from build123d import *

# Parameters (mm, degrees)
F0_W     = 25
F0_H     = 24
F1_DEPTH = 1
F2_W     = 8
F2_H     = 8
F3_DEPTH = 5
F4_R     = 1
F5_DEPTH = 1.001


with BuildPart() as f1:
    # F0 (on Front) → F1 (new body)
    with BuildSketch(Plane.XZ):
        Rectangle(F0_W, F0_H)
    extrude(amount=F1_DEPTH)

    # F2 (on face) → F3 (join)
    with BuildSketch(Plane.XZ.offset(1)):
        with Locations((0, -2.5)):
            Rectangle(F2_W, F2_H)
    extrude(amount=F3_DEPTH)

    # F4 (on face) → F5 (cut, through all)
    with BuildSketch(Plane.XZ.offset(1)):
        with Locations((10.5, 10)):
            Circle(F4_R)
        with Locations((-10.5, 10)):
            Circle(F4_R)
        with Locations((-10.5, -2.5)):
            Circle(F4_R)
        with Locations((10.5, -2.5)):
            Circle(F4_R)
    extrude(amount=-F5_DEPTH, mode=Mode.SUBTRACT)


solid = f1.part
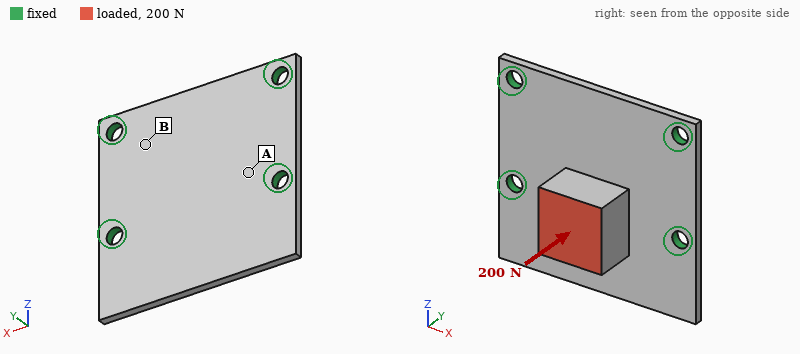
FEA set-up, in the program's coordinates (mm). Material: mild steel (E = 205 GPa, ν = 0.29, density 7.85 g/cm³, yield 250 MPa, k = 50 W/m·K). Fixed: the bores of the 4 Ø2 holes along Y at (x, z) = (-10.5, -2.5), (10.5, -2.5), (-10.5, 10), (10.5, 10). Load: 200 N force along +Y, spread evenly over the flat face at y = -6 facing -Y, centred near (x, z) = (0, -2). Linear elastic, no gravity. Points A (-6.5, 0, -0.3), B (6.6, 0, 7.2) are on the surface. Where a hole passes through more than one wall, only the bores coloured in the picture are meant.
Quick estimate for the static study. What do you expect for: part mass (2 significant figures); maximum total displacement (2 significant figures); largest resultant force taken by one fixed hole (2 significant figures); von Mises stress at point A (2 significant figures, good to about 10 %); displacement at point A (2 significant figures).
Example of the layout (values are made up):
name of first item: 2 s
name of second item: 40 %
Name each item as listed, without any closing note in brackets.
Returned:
part mass: 7.1 g
maximum total displacement: 25 µm
largest resultant force taken by one fixed hole: 100 N
von Mises stress at point A: 45 MPa
displacement at point A: 7.5 µm
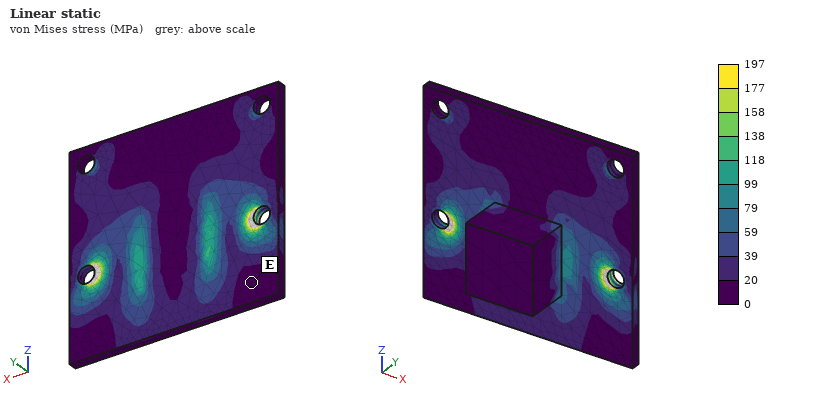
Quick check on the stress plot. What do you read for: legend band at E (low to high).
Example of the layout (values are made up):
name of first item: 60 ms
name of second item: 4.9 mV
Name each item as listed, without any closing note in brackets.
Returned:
legend band at E: 0 to 20 MPa
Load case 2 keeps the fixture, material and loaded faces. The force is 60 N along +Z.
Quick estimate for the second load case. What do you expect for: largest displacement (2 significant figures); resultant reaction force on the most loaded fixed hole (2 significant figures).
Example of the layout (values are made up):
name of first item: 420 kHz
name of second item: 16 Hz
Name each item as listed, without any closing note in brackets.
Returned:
largest displacement: 13 µm
resultant reaction force on the most loaded fixed hole: 21 N
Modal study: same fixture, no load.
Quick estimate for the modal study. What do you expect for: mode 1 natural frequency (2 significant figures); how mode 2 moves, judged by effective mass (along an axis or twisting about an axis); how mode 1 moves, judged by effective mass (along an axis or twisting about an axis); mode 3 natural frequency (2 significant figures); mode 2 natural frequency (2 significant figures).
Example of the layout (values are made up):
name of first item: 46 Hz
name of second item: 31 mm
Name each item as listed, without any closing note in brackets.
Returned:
mode 1 natural frequency: 7200 Hz
how mode 2 moves, judged by effective mass: along Y
how mode 1 moves, judged by effective mass: along Y
mode 3 natural frequency: 14 kHz
mode 2 natural frequency: 10 kHz
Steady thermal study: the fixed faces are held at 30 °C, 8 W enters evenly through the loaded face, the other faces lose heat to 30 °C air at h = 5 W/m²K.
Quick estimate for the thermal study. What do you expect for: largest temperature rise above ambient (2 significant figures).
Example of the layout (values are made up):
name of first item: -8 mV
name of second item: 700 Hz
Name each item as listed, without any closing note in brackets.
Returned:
largest temperature rise above ambient: 55 K
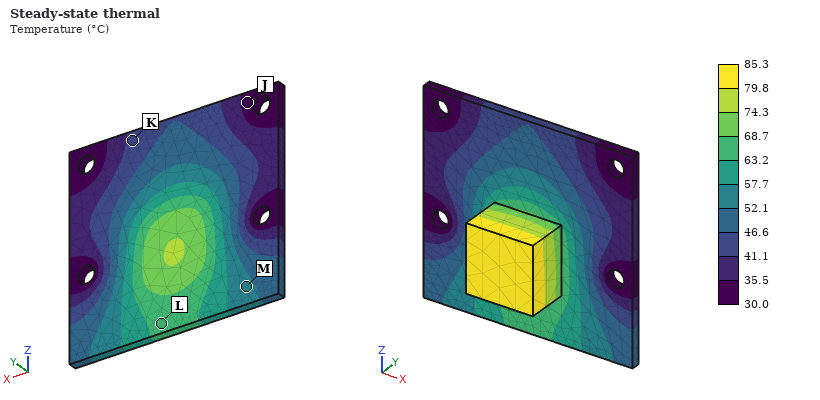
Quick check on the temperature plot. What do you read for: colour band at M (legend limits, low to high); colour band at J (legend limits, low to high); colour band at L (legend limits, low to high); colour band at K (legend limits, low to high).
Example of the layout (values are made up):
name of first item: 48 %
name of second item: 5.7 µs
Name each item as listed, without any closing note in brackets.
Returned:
colour band at M: 52.1 to 57.7 °C
colour band at J: 30.0 to 35.5 °C
colour band at L: 63.2 to 68.7 °C
colour band at K: 41.1 to 46.6 °C
